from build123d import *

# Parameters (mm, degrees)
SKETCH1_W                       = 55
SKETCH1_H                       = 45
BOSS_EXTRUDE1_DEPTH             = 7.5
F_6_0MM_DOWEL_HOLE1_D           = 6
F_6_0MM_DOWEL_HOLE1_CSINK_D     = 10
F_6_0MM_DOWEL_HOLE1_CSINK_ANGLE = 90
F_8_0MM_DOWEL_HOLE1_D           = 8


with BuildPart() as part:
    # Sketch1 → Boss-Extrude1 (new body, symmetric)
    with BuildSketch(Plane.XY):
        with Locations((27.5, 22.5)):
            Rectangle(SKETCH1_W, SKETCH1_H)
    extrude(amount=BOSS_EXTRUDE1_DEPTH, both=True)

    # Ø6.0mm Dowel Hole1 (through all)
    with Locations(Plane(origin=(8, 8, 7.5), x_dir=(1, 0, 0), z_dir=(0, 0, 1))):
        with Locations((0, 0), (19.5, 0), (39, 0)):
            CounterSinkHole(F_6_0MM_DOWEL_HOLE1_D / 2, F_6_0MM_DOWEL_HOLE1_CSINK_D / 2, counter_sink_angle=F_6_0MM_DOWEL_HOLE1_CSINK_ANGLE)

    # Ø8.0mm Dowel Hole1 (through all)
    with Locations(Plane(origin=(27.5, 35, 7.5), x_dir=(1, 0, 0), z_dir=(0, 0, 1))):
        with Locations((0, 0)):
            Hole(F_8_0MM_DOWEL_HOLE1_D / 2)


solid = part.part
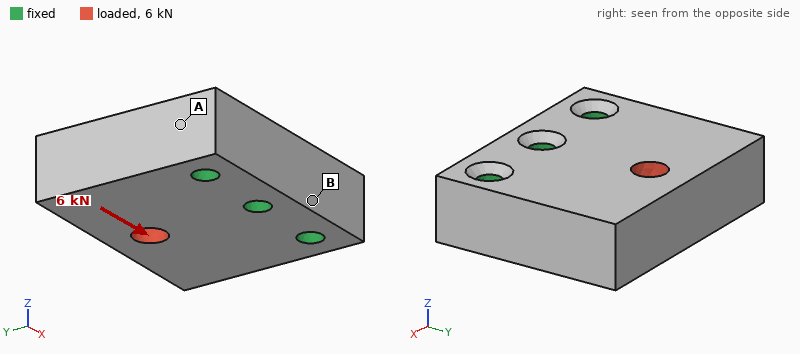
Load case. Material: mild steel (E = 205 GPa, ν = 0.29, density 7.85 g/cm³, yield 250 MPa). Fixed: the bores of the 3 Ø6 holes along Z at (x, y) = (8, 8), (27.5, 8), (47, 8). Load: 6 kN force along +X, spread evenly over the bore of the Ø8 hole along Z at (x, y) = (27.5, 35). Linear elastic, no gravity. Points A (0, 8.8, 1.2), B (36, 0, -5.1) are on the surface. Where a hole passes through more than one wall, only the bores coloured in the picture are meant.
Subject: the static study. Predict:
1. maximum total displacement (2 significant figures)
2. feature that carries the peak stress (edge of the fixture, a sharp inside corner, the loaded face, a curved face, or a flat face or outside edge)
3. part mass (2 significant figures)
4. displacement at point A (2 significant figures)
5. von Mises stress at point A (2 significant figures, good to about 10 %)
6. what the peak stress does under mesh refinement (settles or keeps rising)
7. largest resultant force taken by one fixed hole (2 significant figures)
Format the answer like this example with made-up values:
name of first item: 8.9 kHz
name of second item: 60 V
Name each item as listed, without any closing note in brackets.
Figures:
maximum total displacement: 5.2 µm
feature that carries the peak stress: edge of the fixture
part mass: 270 g
displacement at point A: 0.79 µm
von Mises stress at point A: 14 MPa
what the peak stress does under mesh refinement: keeps rising
largest resultant force taken by one fixed hole: 4.1 kN
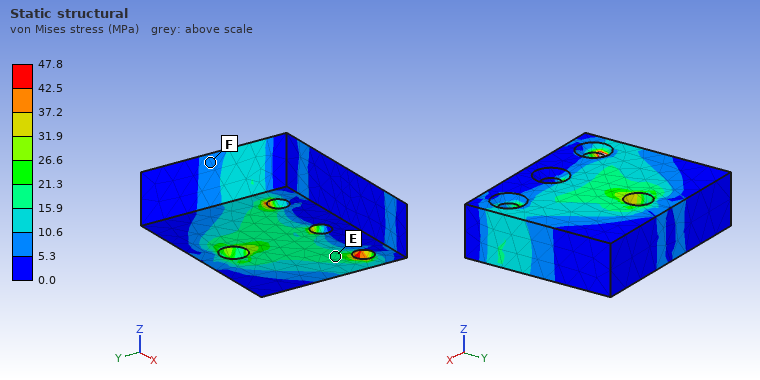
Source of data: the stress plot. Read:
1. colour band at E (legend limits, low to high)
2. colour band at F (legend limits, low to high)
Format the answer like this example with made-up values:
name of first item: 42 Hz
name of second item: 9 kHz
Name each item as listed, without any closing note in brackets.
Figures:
colour band at E: 15.9 to 21.3 MPa
colour band at F: 5.3 to 10.6 MPa
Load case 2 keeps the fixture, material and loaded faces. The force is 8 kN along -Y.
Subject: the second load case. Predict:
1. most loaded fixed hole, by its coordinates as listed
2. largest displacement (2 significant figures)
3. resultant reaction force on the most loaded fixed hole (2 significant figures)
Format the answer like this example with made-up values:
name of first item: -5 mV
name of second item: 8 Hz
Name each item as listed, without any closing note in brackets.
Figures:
most loaded fixed hole, by its coordinates as listed: (27.5, 8)
largest displacement: 3.7 µm
resultant reaction force on the most loaded fixed hole: 3.4 kN
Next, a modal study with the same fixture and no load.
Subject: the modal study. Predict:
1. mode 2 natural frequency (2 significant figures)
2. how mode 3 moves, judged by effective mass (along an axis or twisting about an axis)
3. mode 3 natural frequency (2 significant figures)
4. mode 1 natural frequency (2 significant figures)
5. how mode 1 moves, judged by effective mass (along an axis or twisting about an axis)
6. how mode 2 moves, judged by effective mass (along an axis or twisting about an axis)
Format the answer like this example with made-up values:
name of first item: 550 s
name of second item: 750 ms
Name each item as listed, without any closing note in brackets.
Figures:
mode 2 natural frequency: 13 kHz
how mode 3 moves, judged by effective mass: along X
mode 3 natural frequency: 16 kHz
mode 1 natural frequency: 7900 Hz
how mode 1 moves, judged by effective mass: along Z
how mode 2 moves, judged by effective mass: twisting about Y
